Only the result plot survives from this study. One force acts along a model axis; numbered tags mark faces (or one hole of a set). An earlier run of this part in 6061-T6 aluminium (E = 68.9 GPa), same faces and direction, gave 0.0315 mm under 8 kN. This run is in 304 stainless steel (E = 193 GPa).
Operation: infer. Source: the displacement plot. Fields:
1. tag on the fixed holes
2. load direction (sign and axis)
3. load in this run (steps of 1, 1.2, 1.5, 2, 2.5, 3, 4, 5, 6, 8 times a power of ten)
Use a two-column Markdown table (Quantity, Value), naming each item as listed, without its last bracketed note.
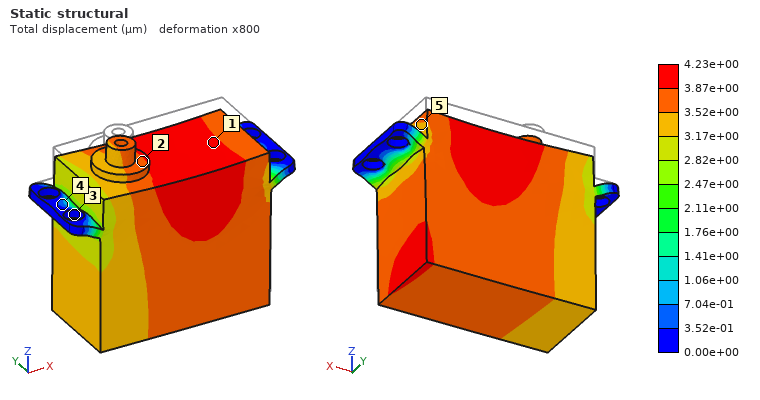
| Quantity | Value |
|---|---|
| tag on the fixed holes | 3 |
| load direction | -Z |
| load in this run | 3 kN |
